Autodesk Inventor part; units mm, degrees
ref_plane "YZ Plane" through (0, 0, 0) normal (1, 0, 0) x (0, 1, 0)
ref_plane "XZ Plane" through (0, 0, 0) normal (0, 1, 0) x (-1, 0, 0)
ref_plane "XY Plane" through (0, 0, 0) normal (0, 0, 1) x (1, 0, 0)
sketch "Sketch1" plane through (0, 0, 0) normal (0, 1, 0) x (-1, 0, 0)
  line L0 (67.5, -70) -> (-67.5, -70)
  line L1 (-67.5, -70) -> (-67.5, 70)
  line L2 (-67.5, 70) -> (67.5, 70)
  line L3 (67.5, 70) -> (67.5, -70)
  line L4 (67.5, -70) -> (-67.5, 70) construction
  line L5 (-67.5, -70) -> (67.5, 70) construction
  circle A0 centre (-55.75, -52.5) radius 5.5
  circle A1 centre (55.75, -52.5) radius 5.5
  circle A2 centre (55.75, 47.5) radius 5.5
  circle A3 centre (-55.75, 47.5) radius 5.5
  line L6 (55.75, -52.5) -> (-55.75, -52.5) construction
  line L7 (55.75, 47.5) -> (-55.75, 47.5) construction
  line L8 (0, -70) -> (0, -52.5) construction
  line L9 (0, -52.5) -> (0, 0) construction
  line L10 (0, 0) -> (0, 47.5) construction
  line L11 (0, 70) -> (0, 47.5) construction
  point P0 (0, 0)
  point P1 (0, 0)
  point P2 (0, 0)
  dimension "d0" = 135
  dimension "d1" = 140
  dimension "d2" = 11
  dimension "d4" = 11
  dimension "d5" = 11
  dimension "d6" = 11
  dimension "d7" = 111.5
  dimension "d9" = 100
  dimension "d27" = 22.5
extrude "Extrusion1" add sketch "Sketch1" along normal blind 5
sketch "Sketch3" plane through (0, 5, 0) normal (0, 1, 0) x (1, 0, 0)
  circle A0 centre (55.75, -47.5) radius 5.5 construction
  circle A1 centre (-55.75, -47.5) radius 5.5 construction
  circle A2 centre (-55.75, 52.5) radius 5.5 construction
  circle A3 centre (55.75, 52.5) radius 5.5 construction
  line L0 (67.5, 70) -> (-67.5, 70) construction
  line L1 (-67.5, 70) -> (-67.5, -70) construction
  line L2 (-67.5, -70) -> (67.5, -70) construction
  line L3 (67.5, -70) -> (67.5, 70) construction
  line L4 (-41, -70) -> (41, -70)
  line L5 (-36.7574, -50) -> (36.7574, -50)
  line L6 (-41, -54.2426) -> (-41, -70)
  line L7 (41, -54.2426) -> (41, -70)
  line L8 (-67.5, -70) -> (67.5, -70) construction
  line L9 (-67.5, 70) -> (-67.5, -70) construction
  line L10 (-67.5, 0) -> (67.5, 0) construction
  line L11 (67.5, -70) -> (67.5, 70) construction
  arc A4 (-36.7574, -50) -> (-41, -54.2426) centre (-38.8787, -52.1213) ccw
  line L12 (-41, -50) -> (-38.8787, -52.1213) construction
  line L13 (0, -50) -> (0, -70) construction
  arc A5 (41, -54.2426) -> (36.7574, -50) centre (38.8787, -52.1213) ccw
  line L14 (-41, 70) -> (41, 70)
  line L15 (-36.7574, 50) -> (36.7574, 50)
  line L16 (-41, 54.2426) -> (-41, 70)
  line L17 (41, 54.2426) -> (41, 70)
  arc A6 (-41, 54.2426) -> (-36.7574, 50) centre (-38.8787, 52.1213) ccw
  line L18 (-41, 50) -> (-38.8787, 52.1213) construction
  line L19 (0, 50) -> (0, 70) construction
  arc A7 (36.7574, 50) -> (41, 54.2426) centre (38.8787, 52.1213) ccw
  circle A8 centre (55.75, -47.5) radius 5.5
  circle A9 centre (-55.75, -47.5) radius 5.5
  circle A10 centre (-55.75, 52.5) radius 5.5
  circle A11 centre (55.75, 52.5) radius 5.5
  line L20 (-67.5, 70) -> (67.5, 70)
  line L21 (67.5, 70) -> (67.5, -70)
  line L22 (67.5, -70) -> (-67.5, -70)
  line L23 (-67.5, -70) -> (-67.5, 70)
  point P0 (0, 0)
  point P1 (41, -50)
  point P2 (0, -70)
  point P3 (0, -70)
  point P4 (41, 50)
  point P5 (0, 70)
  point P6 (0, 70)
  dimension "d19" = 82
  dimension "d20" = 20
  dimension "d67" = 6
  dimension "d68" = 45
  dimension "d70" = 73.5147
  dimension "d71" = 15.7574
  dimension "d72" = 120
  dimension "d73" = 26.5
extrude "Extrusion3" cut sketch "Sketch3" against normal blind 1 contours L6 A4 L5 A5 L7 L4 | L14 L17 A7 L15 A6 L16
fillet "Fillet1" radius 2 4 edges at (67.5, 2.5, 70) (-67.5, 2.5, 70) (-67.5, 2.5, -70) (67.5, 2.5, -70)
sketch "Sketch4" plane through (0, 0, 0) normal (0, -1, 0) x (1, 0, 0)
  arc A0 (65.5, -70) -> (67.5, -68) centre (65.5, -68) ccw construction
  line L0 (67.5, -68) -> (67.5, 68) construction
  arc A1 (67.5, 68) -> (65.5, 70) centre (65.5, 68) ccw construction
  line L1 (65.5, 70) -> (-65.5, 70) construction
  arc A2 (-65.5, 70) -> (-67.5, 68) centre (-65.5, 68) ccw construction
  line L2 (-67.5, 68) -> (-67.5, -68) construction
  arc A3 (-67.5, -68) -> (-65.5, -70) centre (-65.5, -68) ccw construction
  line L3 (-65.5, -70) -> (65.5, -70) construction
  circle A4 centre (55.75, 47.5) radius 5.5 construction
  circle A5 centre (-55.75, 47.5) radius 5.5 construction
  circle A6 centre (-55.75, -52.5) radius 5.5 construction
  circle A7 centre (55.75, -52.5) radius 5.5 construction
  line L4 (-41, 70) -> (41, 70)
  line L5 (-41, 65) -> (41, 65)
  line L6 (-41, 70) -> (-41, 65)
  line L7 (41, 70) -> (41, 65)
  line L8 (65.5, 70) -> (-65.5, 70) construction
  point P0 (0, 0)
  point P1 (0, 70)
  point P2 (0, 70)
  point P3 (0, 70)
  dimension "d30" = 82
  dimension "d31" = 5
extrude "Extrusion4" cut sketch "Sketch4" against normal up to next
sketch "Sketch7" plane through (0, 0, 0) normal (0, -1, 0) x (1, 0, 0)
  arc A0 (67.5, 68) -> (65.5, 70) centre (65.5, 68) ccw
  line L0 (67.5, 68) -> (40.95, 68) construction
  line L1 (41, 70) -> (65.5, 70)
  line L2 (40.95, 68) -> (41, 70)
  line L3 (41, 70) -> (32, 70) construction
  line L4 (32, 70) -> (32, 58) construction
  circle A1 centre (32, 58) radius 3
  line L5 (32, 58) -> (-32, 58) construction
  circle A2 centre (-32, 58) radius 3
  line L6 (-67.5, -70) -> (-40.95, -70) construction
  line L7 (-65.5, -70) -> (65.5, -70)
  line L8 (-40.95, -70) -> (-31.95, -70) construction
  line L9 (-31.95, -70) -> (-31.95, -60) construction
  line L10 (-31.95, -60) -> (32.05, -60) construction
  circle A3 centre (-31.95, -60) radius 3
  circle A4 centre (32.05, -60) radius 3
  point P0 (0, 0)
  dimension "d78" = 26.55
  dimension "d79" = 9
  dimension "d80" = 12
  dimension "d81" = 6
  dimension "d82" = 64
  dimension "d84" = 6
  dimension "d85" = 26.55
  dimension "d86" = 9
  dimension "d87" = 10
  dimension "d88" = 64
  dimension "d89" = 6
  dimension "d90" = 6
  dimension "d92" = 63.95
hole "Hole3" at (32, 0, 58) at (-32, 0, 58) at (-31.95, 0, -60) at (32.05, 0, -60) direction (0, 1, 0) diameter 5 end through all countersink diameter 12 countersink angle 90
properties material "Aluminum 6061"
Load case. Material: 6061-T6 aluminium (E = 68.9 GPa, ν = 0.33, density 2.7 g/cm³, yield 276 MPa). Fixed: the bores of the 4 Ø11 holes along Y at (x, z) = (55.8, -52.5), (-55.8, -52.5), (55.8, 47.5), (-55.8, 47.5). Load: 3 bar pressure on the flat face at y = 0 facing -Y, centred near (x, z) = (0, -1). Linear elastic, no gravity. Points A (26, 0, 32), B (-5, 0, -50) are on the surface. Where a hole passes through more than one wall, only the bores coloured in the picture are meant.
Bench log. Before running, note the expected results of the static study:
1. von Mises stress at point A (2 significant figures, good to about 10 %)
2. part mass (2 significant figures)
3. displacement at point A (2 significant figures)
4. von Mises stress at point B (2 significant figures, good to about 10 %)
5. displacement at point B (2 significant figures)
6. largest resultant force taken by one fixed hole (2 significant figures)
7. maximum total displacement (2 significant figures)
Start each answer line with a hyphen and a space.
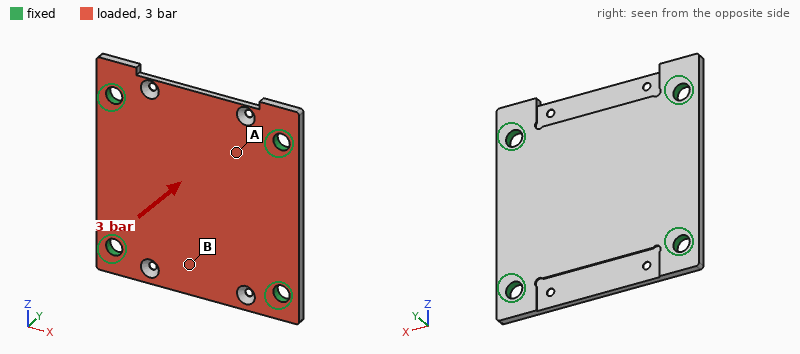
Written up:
- 20 MPa
- 230 g
- 0.16 mm
- 43 MPa
- 0.20 mm
- 1.4 kN
- 0.29 mm
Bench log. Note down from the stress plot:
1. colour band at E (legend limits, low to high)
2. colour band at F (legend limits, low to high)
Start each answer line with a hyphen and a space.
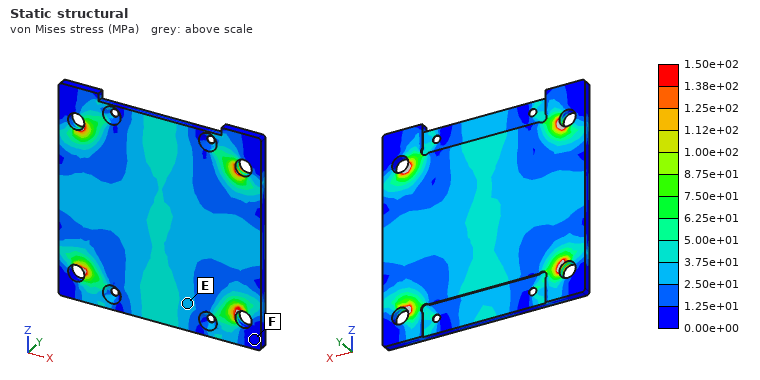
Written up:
- 2.50e+01 to 3.75e+01 MPa
- 0.00e+00 to 1.25e+01 MPa
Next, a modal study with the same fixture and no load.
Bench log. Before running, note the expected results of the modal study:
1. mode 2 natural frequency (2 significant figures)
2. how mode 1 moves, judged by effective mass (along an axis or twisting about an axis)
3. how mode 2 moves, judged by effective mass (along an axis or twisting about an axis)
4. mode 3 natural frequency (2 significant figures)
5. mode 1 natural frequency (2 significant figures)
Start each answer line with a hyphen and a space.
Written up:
- 2500 Hz
- along Y
- twisting about X
- 2900 Hz
- 1700 Hz
